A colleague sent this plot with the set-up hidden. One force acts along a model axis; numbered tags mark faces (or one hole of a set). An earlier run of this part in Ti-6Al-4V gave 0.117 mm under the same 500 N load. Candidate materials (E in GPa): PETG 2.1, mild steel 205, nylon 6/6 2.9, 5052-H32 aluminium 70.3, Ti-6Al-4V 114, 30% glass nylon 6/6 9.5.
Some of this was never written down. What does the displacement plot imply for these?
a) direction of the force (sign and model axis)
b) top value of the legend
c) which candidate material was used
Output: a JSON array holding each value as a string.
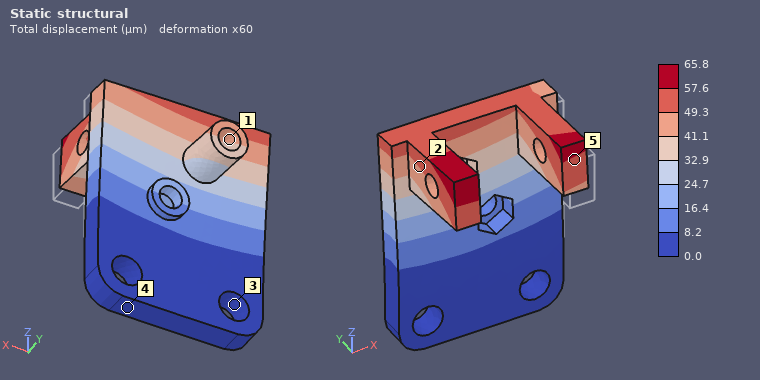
["+Y", "65.8 µm", "mild steel"]
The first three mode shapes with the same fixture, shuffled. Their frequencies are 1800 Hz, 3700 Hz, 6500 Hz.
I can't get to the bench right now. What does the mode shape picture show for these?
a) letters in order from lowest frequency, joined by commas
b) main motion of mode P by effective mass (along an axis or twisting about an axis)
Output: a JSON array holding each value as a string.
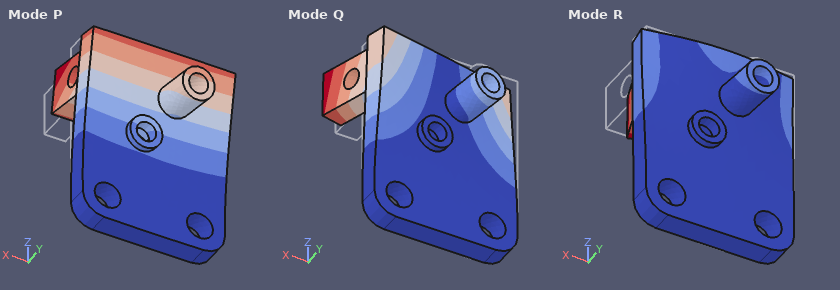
["P, Q, R", "along Y"]
